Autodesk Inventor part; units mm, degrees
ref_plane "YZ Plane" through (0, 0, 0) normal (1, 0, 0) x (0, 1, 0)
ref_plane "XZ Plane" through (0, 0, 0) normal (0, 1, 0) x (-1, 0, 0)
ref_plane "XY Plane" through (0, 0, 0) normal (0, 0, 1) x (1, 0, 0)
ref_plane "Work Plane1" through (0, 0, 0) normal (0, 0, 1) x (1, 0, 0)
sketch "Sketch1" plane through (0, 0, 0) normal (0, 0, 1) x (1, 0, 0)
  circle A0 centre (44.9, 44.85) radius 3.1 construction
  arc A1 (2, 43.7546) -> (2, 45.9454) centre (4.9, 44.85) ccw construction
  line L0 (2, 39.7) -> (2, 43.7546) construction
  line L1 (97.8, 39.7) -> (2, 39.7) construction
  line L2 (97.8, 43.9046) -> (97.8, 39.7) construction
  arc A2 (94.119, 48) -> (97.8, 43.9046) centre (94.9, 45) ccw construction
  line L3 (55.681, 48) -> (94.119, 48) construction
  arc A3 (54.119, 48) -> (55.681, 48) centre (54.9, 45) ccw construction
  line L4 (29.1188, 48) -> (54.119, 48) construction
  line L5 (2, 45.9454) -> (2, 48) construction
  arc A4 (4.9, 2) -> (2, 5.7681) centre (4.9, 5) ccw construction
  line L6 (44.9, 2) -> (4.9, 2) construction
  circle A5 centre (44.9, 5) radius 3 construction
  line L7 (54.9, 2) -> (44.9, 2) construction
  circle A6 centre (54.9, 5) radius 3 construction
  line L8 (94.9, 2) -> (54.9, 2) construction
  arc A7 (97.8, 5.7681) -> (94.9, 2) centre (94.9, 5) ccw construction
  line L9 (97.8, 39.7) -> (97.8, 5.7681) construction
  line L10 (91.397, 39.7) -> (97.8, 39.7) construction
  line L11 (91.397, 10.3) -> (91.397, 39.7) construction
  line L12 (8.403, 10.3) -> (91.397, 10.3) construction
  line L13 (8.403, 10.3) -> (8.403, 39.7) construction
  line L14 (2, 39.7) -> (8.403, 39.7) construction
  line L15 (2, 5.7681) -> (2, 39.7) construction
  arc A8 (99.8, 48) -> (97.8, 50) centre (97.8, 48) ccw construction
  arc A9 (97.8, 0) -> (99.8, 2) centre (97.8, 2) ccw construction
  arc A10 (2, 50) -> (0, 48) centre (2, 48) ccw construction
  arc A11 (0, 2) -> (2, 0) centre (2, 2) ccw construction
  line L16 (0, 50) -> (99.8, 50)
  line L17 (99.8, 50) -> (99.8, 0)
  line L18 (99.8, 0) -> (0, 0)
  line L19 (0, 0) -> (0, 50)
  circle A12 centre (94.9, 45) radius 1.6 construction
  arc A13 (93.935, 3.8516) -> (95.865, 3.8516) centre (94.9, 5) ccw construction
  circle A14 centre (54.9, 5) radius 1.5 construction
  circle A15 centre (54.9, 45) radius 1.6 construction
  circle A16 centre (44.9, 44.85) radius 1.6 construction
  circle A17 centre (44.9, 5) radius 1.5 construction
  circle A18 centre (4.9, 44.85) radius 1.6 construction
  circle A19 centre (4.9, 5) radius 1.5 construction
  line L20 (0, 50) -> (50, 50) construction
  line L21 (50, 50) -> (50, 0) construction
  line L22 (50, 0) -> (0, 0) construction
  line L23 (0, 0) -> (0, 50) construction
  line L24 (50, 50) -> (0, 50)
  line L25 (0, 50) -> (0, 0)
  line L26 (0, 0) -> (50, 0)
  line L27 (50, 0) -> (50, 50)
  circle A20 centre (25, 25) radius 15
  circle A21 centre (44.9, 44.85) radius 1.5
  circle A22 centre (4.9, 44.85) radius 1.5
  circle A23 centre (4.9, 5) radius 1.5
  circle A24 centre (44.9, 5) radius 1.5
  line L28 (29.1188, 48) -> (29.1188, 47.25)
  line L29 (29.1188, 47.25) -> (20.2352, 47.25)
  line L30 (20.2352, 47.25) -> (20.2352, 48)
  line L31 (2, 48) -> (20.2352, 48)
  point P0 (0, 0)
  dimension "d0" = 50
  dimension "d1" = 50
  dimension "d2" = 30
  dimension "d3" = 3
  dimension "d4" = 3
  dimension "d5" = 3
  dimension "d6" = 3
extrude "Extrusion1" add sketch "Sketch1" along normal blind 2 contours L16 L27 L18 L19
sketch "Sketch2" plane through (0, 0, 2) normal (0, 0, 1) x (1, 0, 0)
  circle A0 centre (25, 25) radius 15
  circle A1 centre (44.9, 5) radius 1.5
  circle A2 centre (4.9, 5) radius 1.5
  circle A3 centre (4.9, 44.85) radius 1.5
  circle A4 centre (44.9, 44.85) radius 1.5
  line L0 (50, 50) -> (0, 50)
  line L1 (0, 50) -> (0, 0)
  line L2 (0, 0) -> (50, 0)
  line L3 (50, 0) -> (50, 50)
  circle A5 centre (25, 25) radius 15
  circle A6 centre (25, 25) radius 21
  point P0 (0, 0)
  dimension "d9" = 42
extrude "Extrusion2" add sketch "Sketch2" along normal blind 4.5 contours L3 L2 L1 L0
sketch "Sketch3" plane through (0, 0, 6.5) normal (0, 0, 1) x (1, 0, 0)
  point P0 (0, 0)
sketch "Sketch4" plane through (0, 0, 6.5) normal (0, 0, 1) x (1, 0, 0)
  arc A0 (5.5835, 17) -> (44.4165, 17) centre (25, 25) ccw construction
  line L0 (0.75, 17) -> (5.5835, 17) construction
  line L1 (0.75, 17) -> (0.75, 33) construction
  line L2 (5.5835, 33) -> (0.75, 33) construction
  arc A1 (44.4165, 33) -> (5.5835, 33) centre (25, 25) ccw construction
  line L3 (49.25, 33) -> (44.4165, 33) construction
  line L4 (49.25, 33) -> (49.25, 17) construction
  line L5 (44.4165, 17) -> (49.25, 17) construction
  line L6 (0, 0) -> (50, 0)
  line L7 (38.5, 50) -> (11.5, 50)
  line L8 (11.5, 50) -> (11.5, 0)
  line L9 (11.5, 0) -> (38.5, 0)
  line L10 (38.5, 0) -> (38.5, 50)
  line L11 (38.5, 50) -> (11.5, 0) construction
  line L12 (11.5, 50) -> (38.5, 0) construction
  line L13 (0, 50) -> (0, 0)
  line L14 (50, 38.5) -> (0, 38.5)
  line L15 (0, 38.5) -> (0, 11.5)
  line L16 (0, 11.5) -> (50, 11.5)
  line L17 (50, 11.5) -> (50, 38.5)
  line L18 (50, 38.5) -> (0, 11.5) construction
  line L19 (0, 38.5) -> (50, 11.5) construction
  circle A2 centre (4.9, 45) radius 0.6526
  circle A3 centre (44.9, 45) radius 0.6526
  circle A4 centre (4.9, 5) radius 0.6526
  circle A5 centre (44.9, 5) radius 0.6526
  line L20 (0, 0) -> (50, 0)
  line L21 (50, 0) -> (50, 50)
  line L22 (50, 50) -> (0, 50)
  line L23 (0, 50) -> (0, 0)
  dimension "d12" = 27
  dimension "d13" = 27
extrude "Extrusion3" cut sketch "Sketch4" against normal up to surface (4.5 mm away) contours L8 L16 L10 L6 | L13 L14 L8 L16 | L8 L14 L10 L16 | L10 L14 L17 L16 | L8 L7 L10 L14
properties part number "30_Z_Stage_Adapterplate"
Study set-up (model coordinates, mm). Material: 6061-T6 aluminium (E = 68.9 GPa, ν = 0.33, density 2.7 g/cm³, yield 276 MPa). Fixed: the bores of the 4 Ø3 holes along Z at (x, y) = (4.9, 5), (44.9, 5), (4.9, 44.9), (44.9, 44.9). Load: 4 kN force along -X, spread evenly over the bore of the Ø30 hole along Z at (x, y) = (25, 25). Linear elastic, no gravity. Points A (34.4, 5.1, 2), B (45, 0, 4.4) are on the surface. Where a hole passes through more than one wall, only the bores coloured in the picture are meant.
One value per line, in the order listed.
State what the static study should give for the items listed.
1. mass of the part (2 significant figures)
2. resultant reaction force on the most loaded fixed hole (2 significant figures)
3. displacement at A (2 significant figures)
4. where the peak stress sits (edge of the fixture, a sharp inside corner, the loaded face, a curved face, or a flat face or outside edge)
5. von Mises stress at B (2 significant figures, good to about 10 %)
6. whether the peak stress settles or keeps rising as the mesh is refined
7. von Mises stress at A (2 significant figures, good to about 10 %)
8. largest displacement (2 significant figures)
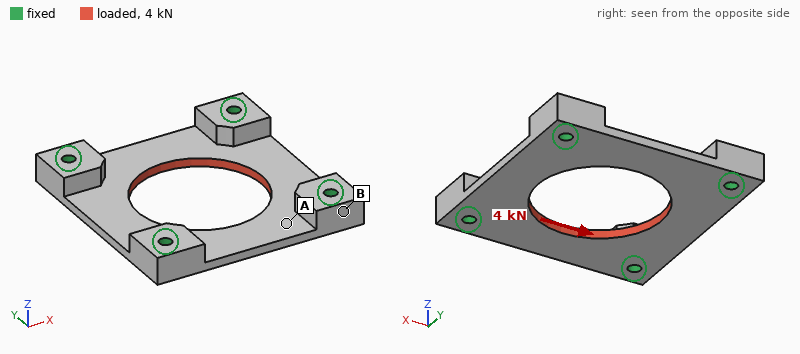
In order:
15 g
1.0 kN
6.1 µm
edge of the fixture
7.6 MPa
keeps rising
35 MPa
22 µm
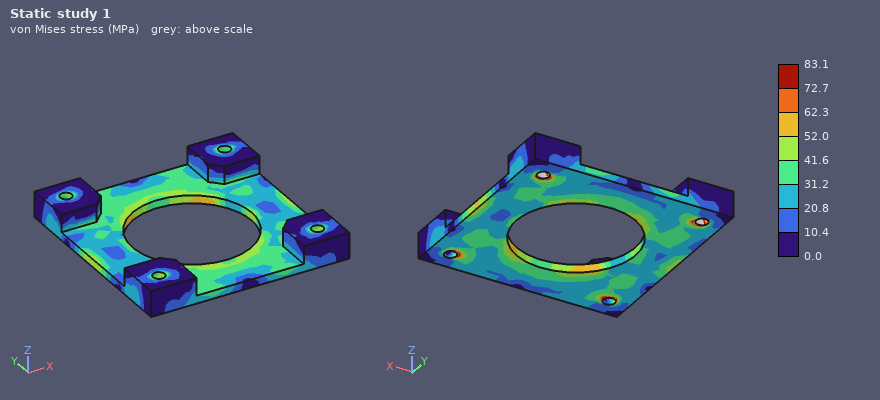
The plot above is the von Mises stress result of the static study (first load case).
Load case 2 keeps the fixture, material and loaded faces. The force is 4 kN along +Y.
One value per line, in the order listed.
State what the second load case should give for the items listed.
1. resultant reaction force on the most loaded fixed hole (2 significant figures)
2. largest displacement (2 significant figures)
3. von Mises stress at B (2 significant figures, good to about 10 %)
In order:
1.0 kN
22 µm
16 MPa
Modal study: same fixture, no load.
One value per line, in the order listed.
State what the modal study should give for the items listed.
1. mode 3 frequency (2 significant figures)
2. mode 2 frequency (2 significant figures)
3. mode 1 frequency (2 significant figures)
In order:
12 kHz
12 kHz
12 kHz
